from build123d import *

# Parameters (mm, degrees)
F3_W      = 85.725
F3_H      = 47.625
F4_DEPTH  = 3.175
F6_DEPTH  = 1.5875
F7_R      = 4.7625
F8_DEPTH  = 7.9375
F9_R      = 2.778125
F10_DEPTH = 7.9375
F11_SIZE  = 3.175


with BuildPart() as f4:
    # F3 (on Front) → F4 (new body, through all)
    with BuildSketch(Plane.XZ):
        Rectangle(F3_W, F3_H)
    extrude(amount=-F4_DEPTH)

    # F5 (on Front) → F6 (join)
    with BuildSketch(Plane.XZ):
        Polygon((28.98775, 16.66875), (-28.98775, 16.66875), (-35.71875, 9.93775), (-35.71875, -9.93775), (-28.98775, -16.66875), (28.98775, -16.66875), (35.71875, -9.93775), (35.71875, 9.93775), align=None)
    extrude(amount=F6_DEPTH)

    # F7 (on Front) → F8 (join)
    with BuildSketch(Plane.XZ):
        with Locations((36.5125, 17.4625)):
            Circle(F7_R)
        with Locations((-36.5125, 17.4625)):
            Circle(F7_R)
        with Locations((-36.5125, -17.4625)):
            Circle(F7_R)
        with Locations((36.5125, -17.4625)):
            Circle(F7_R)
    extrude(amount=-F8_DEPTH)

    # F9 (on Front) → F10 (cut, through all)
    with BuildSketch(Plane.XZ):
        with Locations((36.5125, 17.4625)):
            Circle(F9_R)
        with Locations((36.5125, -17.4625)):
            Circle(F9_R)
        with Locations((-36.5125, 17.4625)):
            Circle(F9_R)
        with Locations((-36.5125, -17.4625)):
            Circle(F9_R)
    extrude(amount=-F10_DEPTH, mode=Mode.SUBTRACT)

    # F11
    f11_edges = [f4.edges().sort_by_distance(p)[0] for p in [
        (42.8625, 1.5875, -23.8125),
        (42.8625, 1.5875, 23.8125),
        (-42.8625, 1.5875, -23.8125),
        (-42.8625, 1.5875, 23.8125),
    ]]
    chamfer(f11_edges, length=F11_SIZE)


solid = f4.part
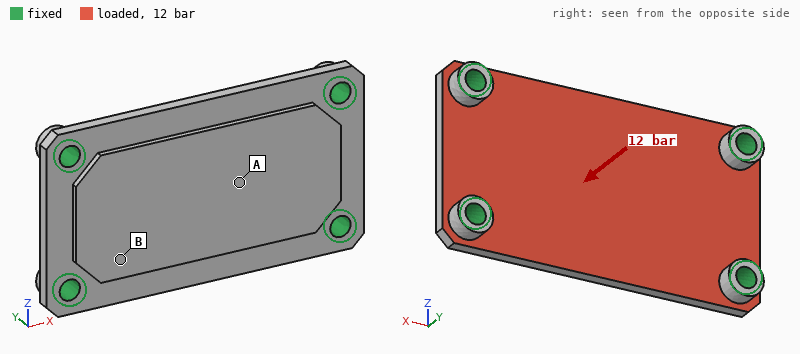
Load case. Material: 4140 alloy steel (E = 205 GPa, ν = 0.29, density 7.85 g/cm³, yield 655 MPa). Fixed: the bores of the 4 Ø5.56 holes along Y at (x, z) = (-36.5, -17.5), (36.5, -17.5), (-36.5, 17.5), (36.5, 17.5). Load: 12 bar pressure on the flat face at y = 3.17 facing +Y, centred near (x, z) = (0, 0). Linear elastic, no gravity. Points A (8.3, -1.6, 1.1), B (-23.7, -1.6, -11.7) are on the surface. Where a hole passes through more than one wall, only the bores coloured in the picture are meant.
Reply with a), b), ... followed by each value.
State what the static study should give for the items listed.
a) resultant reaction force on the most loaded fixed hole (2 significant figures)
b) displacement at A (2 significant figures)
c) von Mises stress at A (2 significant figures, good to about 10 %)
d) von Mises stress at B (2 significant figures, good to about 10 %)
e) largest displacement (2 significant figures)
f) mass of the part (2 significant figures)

a) 1.5 kN
b) 68 µm
c) 83 MPa
d) 47 MPa
e) 83 µm
f) 130 g
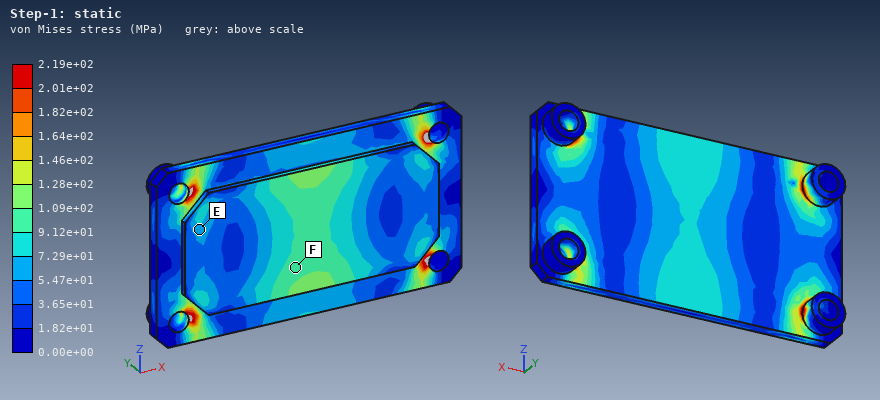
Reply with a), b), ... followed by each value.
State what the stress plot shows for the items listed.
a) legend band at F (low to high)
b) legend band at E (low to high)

a) 9.12e+01 to 1.09e+02 MPa
b) 5.47e+01 to 7.29e+01 MPa
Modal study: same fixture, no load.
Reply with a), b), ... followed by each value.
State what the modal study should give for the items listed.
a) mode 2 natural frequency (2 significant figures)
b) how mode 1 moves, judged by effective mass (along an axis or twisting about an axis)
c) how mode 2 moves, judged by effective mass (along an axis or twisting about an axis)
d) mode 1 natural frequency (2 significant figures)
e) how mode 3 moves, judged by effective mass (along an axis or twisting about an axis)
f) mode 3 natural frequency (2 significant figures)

a) 6200 Hz
b) along Y
c) twisting about X
d) 3900 Hz
e) twisting about Z
f) 11 kHz
